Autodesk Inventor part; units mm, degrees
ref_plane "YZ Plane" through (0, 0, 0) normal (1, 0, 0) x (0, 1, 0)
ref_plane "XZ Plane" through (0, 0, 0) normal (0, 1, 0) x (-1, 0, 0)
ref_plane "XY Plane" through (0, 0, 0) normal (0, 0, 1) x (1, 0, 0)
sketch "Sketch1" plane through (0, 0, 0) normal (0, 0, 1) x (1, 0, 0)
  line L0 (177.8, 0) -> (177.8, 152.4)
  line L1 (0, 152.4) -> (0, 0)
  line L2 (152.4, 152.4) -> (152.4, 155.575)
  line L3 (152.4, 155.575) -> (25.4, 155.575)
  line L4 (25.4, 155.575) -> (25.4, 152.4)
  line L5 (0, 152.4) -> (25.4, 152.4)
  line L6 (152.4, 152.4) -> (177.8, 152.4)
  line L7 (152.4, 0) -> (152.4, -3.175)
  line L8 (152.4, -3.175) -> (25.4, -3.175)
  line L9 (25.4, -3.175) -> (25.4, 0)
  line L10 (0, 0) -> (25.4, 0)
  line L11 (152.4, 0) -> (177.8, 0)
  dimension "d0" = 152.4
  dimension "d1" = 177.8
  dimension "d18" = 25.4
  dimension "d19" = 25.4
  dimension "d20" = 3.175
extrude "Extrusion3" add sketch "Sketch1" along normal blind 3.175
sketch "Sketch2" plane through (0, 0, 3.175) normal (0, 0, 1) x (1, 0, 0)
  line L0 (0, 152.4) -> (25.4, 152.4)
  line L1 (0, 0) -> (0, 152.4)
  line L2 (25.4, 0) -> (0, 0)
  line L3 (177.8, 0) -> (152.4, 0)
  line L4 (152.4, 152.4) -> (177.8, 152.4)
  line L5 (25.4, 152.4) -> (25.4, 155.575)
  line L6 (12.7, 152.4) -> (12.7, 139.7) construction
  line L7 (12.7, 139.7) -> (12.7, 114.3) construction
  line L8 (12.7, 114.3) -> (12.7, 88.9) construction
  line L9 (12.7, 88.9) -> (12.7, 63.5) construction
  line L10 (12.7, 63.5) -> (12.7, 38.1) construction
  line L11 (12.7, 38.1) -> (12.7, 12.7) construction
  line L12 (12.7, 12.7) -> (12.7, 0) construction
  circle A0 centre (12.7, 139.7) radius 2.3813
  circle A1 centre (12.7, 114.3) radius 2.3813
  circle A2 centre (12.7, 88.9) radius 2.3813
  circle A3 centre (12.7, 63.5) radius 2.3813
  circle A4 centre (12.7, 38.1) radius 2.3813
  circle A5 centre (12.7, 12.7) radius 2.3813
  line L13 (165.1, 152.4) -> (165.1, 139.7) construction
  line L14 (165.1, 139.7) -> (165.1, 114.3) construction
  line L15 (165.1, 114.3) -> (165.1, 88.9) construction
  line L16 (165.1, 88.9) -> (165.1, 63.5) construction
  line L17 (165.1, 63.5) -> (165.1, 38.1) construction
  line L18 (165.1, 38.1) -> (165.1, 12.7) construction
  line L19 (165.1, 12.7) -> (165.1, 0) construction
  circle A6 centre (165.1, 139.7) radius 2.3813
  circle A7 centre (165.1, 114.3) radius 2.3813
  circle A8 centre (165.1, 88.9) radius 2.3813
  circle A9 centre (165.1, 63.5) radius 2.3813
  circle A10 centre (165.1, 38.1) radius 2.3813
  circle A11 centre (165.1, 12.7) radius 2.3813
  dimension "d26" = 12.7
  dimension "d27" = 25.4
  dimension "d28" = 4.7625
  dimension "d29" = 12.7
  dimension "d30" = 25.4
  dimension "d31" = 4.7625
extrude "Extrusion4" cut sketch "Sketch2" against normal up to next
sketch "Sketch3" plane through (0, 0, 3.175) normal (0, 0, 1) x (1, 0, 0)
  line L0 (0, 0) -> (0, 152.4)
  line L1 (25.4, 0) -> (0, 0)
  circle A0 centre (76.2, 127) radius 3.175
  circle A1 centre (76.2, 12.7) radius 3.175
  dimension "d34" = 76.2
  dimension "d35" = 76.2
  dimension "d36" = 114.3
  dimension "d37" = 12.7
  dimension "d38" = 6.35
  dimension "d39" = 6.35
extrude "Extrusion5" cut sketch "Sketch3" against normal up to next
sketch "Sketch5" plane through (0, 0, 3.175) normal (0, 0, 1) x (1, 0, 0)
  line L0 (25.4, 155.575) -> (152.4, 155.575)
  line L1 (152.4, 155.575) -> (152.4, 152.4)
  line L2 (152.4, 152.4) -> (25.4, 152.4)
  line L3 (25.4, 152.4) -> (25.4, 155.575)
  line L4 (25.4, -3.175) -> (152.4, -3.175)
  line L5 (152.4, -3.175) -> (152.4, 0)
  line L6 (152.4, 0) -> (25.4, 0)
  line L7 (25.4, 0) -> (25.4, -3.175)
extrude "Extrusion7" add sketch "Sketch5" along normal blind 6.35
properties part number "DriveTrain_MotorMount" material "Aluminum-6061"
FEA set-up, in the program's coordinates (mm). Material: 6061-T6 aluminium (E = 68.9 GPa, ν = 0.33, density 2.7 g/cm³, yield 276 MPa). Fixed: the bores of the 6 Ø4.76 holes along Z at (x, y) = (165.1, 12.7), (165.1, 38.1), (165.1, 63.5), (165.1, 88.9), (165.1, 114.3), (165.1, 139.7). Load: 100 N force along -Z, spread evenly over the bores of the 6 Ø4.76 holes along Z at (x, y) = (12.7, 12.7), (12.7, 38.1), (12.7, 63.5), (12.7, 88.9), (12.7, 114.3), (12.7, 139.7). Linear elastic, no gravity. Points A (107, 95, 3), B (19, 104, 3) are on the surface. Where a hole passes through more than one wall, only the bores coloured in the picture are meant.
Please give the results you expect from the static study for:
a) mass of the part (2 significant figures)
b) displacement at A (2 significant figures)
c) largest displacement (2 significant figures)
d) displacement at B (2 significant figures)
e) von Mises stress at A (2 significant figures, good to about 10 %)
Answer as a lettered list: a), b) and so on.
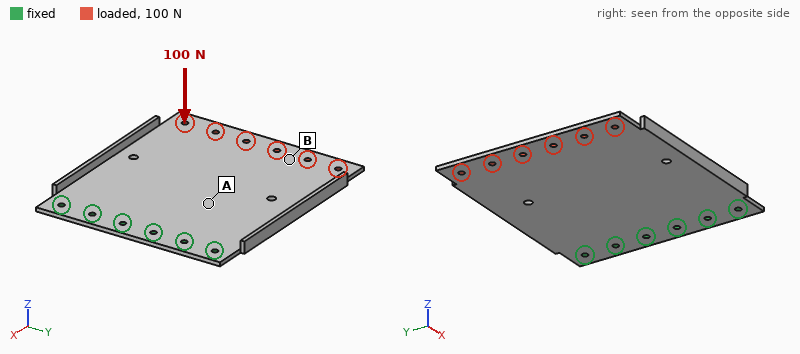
a) 250 g
b) 0.58 mm
c) 2.9 mm
d) 2.4 mm
e) 17 MPa
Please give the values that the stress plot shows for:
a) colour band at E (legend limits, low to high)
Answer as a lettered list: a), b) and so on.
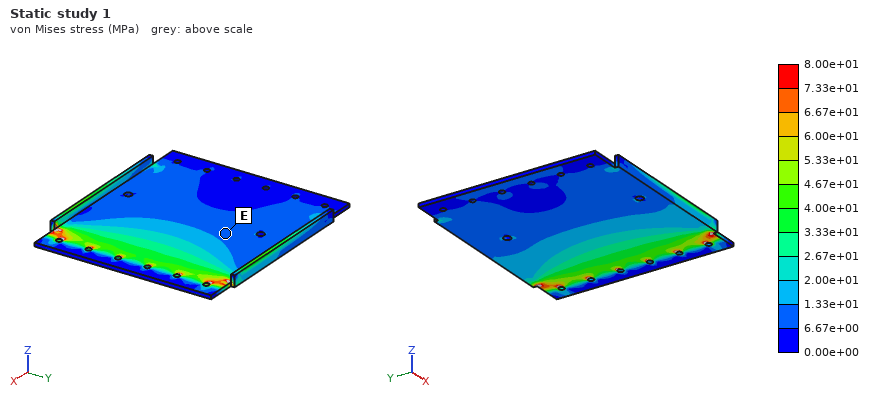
a) 6.67e+00 to 1.33e+01 MPa
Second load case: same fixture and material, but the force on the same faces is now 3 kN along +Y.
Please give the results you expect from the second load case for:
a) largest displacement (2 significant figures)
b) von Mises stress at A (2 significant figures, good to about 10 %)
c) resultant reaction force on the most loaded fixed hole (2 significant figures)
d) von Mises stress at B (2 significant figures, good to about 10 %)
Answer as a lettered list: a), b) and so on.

a) 0.14 mm
b) 16 MPa
c) 2.9 kN
d) 14 MPa
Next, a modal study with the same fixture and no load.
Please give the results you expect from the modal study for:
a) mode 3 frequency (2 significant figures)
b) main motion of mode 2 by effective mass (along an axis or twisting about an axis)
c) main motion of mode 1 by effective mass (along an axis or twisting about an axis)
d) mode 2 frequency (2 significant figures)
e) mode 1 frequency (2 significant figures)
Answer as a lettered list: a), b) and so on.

a) 730 Hz
b) twisting about X
c) along Z
d) 250 Hz
e) 120 Hz
